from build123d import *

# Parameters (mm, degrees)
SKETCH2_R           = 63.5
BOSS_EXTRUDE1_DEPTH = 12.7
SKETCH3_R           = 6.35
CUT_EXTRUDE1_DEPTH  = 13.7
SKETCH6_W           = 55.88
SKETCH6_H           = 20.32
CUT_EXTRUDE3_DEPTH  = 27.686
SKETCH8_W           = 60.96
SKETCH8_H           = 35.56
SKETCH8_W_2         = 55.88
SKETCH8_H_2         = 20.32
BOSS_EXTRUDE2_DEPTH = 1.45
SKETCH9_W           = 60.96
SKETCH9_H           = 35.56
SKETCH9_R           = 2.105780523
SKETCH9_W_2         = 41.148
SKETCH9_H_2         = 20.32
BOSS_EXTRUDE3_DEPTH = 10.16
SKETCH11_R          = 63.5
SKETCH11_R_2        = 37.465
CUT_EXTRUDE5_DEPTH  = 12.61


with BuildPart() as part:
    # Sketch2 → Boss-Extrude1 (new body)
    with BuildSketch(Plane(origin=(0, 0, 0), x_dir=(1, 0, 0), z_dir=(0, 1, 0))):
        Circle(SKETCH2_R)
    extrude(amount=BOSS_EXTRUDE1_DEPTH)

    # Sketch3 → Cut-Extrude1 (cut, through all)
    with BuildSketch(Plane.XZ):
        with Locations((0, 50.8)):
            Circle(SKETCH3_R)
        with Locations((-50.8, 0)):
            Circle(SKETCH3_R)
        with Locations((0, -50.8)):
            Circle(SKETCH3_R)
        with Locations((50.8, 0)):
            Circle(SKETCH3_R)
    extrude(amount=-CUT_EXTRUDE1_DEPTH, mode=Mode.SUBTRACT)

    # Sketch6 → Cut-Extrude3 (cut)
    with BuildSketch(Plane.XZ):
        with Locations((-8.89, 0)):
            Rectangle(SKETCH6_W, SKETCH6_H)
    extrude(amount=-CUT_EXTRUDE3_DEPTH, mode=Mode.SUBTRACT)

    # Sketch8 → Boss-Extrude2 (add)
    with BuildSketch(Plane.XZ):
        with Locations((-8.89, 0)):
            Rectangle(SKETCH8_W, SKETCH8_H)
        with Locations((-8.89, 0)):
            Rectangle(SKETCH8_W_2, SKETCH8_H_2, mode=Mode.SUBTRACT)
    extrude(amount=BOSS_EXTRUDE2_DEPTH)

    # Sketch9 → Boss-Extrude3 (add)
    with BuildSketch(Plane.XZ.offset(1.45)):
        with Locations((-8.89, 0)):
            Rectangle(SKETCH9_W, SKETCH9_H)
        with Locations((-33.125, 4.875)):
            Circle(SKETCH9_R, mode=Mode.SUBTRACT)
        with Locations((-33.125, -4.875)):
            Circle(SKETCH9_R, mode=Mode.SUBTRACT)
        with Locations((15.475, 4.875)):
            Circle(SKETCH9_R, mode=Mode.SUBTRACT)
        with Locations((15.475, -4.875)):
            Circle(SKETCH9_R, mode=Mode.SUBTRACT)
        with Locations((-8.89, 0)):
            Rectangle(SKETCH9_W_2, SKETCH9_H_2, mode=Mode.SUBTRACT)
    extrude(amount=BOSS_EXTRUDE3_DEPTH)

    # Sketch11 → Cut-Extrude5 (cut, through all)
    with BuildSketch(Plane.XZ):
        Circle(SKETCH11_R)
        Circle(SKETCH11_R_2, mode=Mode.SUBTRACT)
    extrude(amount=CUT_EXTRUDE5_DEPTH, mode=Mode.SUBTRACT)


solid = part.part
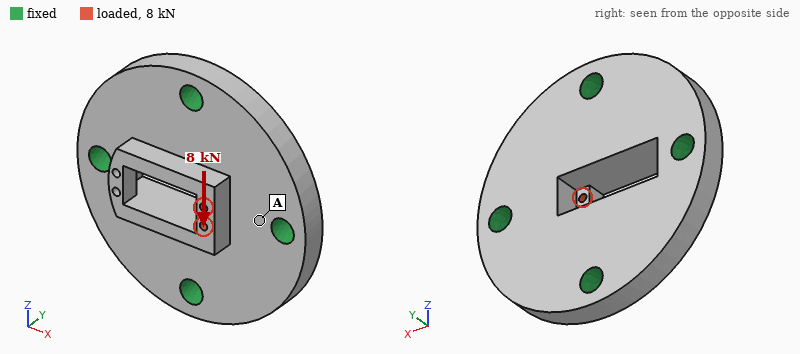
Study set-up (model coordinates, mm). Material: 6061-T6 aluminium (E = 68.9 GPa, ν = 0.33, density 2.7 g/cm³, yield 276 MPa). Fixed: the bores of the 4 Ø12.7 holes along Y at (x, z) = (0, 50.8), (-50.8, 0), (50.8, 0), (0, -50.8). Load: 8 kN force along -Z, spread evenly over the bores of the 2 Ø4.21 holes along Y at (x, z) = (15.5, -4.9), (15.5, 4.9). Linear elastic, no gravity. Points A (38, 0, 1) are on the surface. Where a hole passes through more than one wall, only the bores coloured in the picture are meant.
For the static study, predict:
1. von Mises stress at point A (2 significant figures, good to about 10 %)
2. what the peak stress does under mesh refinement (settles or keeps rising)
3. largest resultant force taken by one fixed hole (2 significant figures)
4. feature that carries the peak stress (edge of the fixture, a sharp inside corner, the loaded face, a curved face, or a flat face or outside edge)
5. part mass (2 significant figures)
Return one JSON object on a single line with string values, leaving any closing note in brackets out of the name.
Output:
{"von Mises stress at point A": "11 MPa", "what the peak stress does under mesh refinement": "keeps rising", "largest resultant force taken by one fixed hole": "3.0 kN", "feature that carries the peak stress": "a sharp inside corner", "part mass": "410 g"}
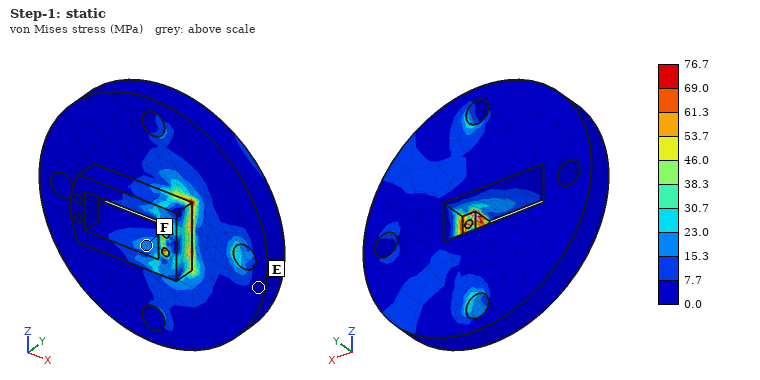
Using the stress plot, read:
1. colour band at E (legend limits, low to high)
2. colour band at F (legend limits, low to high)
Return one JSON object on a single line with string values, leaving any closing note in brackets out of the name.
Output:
{"colour band at E": "0.0 to 7.7 MPa", "colour band at F": "15.3 to 23.0 MPa"}
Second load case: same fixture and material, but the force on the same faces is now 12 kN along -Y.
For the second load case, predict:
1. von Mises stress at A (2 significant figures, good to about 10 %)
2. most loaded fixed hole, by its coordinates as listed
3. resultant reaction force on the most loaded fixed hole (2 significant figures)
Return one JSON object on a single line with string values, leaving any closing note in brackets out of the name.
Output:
{"von Mises stress at A": "36 MPa", "most loaded fixed hole, by its coordinates as listed": "(50.8, 0)", "resultant reaction force on the most loaded fixed hole": "5.9 kN"}
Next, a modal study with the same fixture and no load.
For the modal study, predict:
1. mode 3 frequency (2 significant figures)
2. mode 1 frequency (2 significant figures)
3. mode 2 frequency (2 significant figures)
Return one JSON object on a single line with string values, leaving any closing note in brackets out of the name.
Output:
{"mode 3 frequency": "9900 Hz", "mode 1 frequency": "9400 Hz", "mode 2 frequency": "9600 Hz"}
